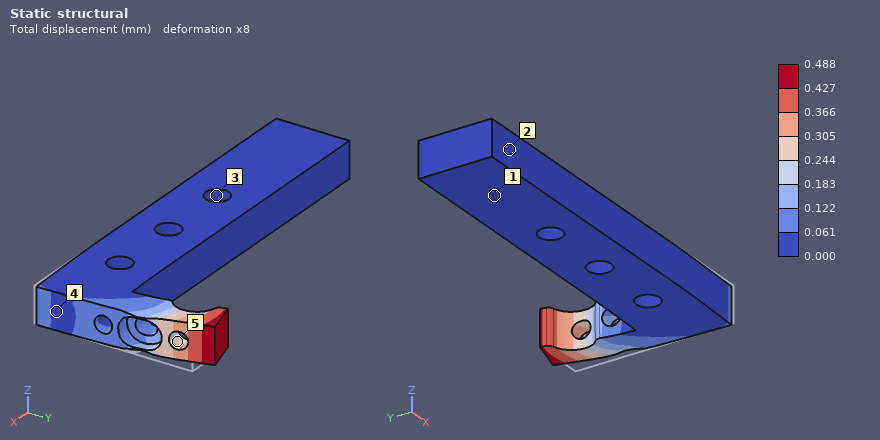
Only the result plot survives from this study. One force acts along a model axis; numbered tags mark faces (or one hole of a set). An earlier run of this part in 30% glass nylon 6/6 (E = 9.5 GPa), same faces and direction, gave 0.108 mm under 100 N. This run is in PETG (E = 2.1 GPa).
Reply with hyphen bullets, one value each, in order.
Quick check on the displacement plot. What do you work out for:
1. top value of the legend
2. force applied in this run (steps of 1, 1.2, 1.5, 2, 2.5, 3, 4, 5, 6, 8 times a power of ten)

- 0.488 mm
- 100 N
